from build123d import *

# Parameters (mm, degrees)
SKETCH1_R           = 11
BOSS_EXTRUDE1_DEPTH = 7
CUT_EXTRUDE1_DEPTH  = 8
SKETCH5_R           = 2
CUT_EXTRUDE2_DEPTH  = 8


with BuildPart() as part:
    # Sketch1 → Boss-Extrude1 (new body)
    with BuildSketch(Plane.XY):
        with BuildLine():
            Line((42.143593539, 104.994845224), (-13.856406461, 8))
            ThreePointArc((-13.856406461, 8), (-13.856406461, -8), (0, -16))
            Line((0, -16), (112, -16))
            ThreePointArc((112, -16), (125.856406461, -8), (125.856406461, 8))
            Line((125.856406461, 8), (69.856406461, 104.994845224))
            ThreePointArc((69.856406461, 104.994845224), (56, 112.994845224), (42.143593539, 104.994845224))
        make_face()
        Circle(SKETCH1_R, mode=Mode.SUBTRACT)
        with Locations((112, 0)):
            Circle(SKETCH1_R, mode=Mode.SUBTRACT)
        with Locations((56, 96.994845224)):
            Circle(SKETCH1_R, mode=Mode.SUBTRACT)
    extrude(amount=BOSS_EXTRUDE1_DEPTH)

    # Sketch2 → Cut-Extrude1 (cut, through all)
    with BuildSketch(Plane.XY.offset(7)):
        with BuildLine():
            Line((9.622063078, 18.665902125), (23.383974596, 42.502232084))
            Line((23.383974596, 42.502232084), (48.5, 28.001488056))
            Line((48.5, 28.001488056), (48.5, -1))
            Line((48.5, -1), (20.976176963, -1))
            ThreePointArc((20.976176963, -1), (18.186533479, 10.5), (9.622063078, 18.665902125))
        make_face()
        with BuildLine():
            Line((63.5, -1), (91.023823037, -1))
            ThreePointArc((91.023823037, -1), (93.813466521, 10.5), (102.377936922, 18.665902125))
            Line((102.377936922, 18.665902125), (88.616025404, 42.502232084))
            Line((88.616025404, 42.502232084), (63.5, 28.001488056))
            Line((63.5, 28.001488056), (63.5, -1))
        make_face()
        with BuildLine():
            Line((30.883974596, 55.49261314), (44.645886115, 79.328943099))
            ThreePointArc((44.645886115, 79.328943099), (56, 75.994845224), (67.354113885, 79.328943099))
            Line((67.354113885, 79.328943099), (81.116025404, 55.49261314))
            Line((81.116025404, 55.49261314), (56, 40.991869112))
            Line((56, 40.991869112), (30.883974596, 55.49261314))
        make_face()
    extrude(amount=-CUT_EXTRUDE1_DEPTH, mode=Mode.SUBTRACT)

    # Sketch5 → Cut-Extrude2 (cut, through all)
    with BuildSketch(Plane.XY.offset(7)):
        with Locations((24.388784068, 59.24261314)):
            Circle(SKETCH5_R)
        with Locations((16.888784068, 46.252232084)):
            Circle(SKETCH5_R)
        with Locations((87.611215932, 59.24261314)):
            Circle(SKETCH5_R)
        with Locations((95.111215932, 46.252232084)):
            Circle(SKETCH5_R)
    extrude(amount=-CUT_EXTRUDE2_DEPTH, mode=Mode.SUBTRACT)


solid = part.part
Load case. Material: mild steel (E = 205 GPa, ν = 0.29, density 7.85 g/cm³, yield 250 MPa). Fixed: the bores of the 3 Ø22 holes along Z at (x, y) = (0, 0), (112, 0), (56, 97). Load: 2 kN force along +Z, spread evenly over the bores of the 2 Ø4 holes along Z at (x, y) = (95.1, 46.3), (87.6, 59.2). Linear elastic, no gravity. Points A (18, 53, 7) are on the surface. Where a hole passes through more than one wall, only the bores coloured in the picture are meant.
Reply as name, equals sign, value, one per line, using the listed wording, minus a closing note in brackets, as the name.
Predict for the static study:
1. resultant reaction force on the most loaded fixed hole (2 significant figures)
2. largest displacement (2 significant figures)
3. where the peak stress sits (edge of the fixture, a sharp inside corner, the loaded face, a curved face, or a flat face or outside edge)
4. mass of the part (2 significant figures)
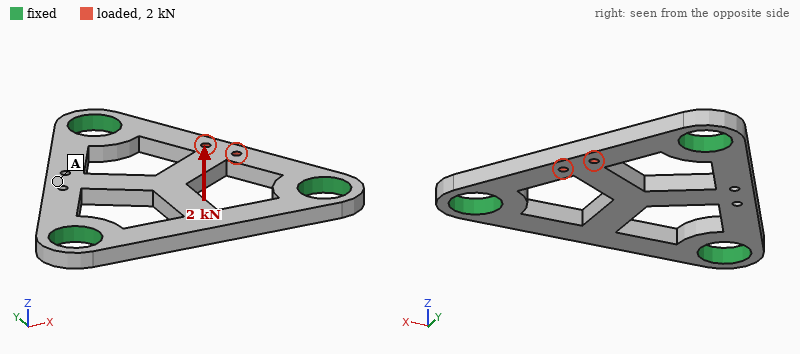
resultant reaction force on the most loaded fixed hole = 1.0 kN
largest displacement = 88 µm
where the peak stress sits = the loaded face
mass of the part = 380 g
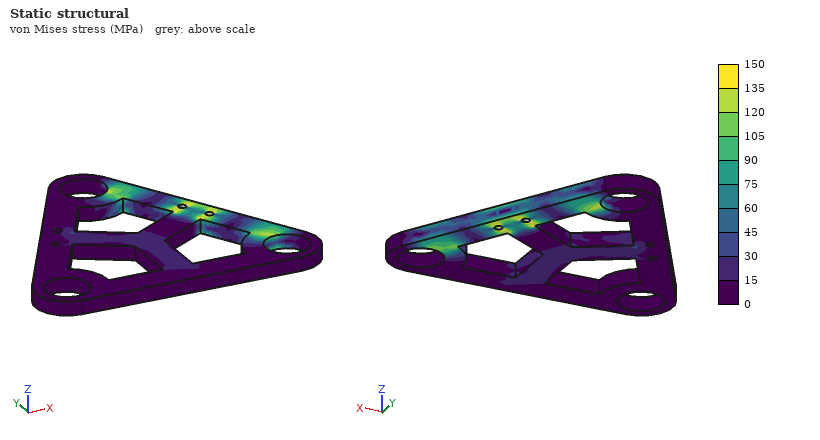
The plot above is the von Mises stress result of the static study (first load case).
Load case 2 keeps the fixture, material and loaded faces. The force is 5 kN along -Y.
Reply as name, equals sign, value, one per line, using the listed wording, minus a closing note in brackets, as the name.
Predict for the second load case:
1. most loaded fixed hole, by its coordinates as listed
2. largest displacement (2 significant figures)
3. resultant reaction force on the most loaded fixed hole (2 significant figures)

most loaded fixed hole, by its coordinates as listed = (112, 0)
largest displacement = 12 µm
resultant reaction force on the most loaded fixed hole = 2.5 kN
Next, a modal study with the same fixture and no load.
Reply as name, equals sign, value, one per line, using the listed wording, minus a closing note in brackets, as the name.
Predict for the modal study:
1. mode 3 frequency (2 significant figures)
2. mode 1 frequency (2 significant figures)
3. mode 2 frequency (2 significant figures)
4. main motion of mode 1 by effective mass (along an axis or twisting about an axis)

mode 3 frequency = 4200 Hz
mode 1 frequency = 2900 Hz
mode 2 frequency = 4200 Hz
main motion of mode 1 by effective mass = along Z
